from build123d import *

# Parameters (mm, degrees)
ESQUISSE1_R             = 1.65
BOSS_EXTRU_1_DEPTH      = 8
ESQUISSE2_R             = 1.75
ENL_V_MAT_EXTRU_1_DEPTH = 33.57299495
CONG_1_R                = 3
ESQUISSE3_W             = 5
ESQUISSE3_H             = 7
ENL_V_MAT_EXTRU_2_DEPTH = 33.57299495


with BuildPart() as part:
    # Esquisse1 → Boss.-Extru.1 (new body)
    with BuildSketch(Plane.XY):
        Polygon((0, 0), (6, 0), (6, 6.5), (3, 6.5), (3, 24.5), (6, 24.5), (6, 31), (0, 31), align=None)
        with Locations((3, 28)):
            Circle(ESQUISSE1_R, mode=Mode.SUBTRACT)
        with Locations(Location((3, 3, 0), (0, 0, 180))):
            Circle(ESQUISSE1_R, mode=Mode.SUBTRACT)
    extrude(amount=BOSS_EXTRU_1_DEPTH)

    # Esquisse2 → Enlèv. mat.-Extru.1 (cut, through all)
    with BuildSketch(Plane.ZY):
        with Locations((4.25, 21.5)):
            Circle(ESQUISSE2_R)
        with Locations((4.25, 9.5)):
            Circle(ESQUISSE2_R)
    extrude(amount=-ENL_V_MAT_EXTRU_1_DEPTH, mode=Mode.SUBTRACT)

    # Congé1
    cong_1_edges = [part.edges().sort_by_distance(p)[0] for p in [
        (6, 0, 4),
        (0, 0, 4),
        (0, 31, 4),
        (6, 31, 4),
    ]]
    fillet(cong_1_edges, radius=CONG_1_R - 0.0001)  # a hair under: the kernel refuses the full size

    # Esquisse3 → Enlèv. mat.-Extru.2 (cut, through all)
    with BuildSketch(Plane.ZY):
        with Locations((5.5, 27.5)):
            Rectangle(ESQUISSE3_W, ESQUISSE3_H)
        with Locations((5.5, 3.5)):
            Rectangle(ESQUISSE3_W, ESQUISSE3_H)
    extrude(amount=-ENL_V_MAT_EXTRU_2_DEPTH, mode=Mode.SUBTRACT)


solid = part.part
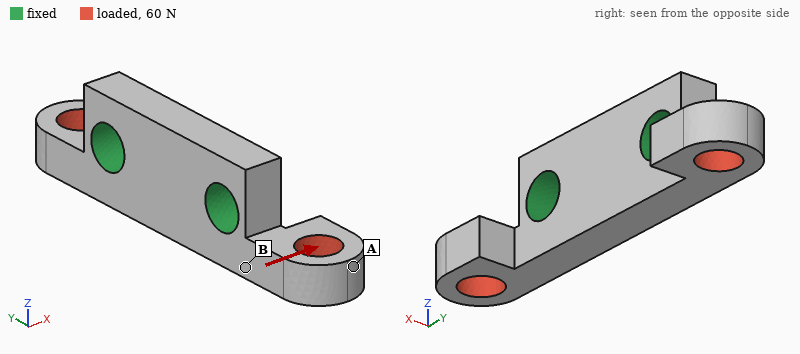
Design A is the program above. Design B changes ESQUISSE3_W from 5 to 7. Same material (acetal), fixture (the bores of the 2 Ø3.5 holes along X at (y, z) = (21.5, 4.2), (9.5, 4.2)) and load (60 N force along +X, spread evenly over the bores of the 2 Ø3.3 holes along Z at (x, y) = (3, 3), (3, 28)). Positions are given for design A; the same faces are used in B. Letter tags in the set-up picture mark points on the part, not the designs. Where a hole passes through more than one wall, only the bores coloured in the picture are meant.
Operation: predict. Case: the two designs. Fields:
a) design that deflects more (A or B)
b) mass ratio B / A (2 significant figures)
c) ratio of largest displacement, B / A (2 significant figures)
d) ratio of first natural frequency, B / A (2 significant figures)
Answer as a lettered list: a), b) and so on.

a) B
b) 0.89
c) 1.6
d) 0.89
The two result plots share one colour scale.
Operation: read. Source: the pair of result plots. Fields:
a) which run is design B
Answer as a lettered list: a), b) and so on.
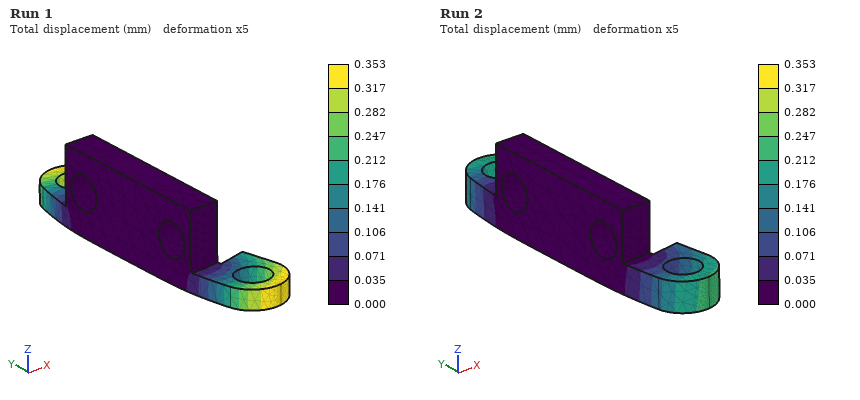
a) Run 1
